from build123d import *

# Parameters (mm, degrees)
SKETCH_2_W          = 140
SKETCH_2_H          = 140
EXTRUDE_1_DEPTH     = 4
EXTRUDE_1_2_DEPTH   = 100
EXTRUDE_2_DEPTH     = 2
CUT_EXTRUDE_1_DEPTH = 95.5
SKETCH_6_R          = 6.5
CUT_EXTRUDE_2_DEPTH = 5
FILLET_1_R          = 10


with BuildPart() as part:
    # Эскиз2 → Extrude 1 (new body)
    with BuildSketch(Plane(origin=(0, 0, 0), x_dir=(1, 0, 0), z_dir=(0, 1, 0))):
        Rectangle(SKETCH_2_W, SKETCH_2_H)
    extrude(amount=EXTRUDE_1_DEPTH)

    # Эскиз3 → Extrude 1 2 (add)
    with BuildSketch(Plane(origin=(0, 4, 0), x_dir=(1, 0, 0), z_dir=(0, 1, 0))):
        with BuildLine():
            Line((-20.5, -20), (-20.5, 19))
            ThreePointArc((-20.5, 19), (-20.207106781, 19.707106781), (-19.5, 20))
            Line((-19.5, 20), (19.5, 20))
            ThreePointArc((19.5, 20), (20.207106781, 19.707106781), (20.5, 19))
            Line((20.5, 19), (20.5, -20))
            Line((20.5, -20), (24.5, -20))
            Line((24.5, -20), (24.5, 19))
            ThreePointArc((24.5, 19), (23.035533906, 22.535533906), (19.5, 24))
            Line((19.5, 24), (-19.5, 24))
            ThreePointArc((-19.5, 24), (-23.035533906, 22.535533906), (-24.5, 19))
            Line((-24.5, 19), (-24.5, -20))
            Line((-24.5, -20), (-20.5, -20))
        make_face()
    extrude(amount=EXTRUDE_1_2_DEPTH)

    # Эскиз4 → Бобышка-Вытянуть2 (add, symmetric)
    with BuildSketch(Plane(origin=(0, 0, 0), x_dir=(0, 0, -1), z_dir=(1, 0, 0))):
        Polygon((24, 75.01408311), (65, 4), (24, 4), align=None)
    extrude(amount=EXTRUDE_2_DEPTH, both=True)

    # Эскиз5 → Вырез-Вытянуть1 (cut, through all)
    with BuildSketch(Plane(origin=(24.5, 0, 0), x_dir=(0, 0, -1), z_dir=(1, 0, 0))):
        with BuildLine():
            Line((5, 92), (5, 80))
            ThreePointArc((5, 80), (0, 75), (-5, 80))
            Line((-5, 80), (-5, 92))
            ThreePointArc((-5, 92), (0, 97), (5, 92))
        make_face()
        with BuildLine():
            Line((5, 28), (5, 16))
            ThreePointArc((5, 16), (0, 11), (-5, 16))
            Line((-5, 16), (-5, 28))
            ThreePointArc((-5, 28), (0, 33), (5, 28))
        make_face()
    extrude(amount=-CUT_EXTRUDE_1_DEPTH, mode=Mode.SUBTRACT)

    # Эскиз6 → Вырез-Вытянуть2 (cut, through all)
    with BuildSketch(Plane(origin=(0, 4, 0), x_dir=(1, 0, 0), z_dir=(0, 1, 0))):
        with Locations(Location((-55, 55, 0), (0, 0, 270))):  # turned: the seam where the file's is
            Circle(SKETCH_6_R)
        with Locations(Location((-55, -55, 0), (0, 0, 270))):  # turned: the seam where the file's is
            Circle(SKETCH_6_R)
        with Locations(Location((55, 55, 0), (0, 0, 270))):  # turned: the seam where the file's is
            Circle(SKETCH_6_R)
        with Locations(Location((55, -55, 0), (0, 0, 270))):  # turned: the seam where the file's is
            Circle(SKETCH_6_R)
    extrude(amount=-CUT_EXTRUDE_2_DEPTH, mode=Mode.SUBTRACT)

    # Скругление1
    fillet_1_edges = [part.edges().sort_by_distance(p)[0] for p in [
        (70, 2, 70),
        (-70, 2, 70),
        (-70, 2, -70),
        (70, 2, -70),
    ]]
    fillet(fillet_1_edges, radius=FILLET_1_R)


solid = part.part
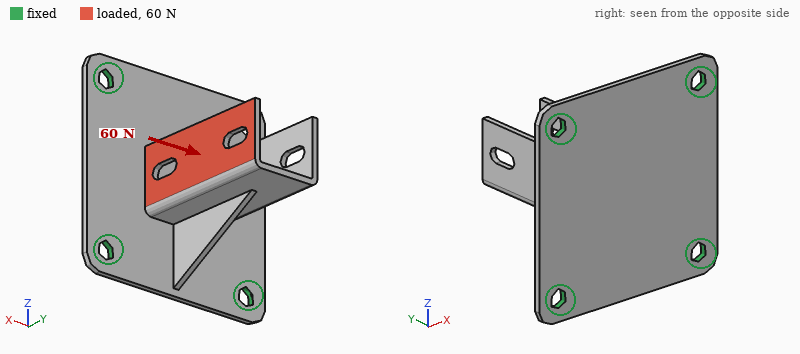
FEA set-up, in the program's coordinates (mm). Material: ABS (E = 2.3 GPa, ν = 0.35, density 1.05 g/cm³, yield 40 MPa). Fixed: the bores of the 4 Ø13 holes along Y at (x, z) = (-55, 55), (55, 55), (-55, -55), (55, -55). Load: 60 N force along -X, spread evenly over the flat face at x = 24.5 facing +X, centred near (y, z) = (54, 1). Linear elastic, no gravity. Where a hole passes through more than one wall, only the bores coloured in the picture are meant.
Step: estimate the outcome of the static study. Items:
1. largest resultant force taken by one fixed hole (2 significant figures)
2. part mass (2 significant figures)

32 N
140 g
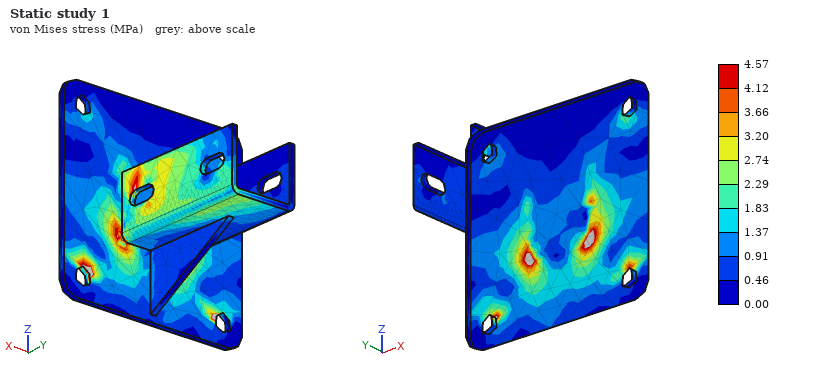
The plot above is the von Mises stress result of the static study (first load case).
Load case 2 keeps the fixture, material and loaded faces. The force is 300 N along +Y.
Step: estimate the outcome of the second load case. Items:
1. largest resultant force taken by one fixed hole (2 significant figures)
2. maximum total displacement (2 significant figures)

120 N
2.5 mm
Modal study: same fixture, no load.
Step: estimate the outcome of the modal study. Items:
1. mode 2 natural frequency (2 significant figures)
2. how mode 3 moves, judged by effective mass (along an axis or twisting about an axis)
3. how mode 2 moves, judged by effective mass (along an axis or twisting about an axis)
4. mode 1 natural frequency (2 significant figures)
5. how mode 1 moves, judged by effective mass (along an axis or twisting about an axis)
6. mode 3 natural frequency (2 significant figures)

250 Hz
along Y
along Z
190 Hz
along X
300 Hz
